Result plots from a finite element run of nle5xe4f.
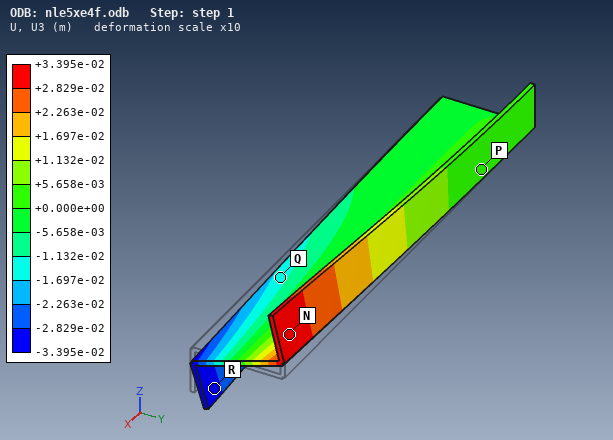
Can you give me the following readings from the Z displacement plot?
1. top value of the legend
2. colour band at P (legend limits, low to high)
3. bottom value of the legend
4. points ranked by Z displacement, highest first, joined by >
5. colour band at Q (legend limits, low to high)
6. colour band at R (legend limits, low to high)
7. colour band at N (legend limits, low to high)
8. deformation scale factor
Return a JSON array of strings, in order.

["+3.395e-02 m", "+0.000e+00 to +5.658e-03 m", "-3.395e-02 m", "N > P > Q > R", "-1.697e-02 to -1.132e-02 m", "-3.395e-02 to -2.829e-02 m", "+2.829e-02 to +3.395e-02 m", "10"]
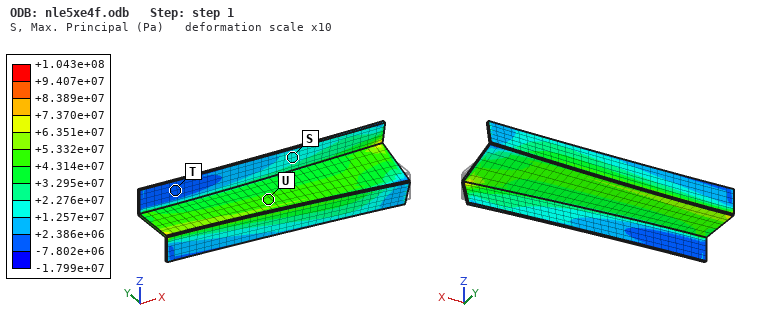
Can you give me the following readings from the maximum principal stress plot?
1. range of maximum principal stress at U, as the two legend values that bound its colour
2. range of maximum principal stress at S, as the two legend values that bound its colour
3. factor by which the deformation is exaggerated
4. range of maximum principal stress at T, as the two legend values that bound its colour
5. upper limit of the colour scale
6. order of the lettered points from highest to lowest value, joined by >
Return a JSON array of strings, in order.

["+4.314e+07 to +5.332e+07 Pa", "+1.257e+07 to +2.276e+07 Pa", "10", "-7.802e+06 to +2.386e+06 Pa", "+1.043e+08 Pa", "U > S > T"]
